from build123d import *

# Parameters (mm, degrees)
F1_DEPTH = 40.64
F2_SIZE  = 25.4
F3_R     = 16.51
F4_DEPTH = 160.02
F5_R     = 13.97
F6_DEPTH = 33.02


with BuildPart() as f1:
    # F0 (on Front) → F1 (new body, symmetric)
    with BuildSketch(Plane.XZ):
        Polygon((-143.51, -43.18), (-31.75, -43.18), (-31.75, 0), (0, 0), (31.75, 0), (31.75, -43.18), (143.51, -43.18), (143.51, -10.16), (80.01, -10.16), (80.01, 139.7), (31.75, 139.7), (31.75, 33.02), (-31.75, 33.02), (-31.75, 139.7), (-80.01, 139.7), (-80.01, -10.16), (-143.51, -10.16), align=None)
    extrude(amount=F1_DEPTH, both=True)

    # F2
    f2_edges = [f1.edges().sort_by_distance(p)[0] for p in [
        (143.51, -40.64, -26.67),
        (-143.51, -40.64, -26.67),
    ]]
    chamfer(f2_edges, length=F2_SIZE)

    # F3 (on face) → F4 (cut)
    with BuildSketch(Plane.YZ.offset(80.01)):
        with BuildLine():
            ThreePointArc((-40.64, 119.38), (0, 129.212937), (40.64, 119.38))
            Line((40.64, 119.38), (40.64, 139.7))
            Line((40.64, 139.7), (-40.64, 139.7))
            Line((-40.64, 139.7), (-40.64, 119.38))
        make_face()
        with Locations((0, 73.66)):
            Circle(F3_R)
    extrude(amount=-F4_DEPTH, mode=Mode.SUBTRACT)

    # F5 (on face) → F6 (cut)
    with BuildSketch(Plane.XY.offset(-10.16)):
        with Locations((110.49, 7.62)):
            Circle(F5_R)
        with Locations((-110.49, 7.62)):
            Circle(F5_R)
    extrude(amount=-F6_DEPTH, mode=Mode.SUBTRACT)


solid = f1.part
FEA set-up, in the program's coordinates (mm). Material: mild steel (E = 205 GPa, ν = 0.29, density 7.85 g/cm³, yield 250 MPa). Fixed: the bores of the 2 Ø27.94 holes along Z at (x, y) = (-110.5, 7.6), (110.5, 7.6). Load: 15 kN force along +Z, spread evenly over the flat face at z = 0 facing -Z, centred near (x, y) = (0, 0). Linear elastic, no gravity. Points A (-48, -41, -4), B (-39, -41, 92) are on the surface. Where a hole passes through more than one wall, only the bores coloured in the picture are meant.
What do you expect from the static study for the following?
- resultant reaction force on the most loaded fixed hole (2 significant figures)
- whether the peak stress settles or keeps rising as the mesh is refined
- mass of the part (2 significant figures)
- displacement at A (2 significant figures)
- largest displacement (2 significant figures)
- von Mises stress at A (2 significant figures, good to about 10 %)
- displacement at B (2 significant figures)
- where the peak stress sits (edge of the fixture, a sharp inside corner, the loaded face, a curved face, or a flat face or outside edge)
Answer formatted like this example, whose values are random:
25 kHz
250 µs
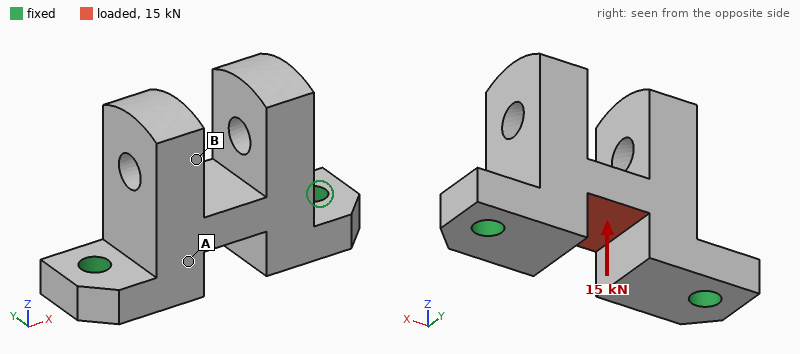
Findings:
11 kN
keeps rising
13 kg
5.0 µm
9.2 µm
3.9 MPa
7.6 µm
edge of the fixture
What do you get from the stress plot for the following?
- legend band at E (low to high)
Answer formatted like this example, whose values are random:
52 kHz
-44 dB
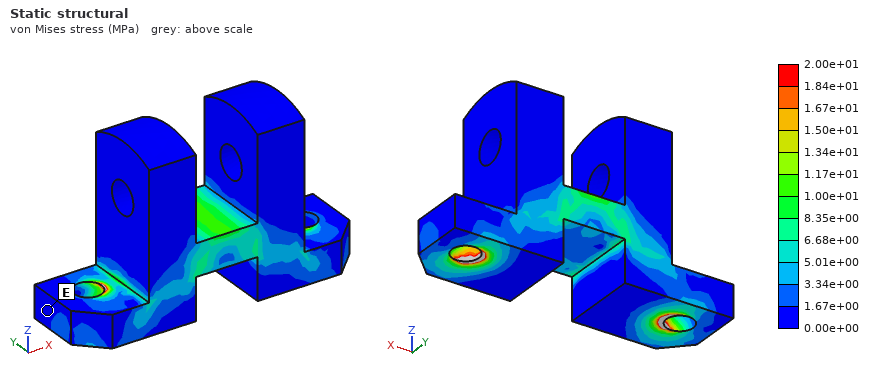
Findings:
0.00e+00 to 1.67e+00 MPa
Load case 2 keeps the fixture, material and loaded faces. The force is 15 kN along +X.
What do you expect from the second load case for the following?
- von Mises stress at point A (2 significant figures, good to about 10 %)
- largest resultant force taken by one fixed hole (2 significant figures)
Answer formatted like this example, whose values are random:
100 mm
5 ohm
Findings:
4.8 MPa
7.7 kN
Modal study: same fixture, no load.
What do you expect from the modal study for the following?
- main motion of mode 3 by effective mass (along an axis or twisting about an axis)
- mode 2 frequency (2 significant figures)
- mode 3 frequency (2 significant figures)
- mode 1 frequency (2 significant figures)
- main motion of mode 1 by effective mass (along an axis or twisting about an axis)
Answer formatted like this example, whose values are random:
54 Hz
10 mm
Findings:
along X
1700 Hz
2000 Hz
1000 Hz
along Y
